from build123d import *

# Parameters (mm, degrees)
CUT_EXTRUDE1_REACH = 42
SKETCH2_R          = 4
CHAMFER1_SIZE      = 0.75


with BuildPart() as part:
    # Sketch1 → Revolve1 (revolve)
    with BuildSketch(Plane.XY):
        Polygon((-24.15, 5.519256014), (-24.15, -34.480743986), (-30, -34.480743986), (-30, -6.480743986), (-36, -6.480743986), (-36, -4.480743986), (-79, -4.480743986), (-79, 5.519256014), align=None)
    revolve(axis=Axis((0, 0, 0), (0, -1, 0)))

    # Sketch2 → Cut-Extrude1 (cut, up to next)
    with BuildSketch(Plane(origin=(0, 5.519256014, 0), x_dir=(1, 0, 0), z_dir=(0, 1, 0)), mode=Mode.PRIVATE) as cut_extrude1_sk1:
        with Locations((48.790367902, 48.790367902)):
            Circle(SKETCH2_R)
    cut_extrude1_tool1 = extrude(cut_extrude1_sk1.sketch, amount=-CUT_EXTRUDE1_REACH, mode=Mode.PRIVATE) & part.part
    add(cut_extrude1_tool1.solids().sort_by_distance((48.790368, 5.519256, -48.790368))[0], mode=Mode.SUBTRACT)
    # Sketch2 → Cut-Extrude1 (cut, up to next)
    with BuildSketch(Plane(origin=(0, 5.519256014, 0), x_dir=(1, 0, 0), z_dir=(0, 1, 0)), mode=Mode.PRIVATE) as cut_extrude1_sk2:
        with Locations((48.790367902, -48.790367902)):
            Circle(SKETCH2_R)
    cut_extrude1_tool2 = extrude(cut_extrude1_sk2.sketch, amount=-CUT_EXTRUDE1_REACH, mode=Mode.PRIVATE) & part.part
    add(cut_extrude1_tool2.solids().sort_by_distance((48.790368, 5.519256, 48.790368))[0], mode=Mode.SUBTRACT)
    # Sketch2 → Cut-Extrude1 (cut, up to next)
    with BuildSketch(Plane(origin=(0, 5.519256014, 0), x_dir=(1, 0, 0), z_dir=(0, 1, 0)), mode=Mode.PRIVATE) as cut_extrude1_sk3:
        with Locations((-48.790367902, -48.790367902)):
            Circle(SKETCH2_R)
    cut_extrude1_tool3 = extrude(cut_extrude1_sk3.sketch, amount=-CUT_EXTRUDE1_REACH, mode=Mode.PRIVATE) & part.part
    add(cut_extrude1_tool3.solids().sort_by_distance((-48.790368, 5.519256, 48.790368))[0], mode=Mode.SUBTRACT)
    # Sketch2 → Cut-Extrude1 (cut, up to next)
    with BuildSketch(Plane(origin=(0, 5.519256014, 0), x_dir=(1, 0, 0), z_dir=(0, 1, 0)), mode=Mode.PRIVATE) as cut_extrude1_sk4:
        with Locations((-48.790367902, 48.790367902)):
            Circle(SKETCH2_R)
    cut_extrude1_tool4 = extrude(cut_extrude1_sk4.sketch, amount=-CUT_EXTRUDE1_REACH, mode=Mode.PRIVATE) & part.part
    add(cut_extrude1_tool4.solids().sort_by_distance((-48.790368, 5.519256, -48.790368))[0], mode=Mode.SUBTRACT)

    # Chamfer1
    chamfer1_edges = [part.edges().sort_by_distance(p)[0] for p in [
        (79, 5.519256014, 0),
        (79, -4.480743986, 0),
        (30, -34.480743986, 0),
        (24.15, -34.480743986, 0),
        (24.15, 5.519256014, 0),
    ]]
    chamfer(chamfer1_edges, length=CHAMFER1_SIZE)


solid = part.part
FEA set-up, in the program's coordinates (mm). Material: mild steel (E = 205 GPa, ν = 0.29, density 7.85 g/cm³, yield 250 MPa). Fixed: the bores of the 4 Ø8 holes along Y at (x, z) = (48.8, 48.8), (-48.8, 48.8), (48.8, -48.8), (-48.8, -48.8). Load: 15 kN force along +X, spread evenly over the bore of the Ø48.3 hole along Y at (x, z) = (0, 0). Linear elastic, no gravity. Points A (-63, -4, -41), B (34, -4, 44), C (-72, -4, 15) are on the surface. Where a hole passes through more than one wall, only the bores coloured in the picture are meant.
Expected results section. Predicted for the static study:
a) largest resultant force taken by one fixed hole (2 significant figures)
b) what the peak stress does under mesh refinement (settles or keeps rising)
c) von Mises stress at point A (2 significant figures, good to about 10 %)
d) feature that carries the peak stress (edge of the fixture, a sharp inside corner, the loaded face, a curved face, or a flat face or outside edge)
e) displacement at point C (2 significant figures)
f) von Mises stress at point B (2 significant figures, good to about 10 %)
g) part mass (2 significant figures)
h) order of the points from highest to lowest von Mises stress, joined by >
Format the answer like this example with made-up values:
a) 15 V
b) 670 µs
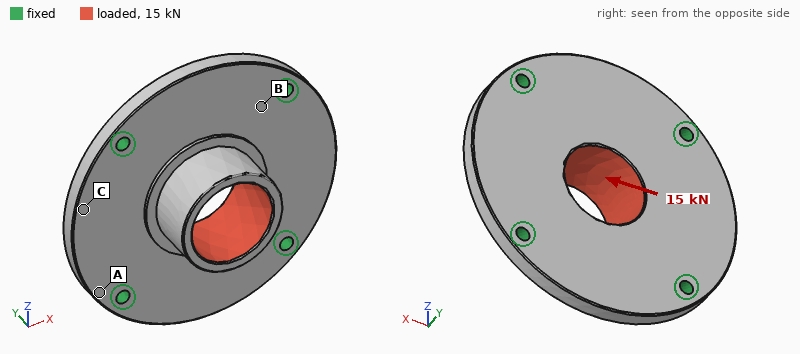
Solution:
a) 4.1 kN
b) keeps rising
c) 11 MPa
d) edge of the fixture
e) 6.2 µm
f) 20 MPa
g) 1.6 kg
h) B > A > C
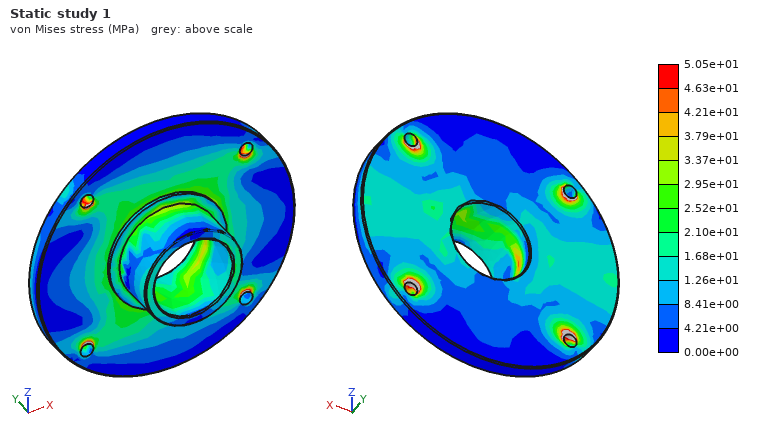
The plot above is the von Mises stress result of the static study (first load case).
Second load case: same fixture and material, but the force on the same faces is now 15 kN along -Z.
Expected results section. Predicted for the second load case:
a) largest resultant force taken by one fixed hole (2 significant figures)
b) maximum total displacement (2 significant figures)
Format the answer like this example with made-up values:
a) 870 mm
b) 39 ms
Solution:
a) 4.1 kN
b) 24 µm
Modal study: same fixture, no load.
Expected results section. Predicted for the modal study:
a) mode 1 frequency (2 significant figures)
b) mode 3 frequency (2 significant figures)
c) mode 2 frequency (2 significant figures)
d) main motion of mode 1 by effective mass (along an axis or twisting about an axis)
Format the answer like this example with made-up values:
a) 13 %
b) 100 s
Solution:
a) 3800 Hz
b) 4400 Hz
c) 4400 Hz
d) along Y
